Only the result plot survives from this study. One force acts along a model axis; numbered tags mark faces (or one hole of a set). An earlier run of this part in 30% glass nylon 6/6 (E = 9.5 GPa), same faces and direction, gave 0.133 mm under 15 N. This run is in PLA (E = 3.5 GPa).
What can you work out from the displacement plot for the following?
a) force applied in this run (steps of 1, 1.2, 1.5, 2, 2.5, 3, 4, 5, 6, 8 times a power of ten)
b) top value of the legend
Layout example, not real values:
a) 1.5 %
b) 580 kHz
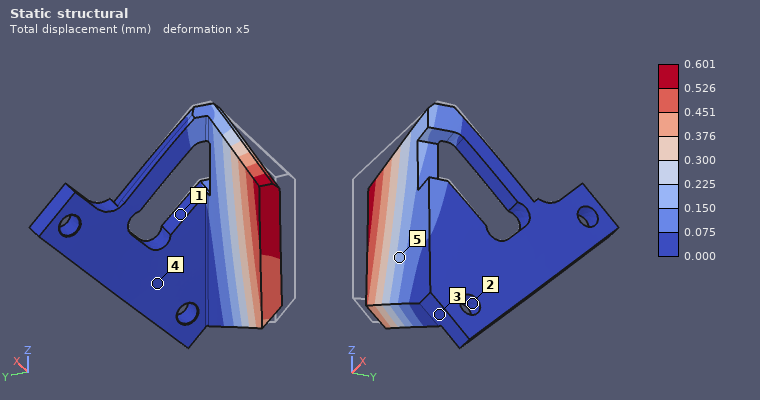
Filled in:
a) 25 N
b) 0.601 mm
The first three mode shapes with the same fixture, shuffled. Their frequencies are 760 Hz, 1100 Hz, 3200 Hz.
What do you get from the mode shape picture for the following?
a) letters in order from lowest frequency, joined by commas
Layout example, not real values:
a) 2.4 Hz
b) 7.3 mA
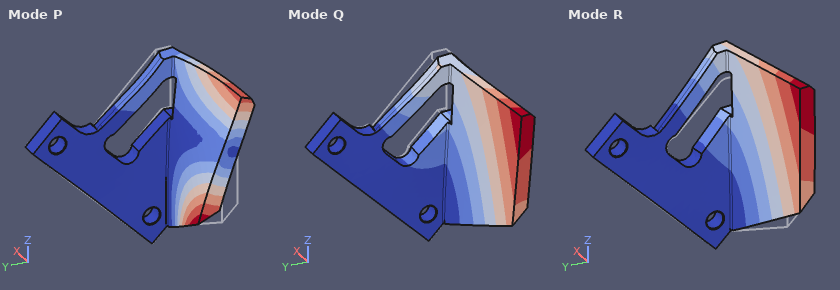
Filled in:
a) R, Q, P
